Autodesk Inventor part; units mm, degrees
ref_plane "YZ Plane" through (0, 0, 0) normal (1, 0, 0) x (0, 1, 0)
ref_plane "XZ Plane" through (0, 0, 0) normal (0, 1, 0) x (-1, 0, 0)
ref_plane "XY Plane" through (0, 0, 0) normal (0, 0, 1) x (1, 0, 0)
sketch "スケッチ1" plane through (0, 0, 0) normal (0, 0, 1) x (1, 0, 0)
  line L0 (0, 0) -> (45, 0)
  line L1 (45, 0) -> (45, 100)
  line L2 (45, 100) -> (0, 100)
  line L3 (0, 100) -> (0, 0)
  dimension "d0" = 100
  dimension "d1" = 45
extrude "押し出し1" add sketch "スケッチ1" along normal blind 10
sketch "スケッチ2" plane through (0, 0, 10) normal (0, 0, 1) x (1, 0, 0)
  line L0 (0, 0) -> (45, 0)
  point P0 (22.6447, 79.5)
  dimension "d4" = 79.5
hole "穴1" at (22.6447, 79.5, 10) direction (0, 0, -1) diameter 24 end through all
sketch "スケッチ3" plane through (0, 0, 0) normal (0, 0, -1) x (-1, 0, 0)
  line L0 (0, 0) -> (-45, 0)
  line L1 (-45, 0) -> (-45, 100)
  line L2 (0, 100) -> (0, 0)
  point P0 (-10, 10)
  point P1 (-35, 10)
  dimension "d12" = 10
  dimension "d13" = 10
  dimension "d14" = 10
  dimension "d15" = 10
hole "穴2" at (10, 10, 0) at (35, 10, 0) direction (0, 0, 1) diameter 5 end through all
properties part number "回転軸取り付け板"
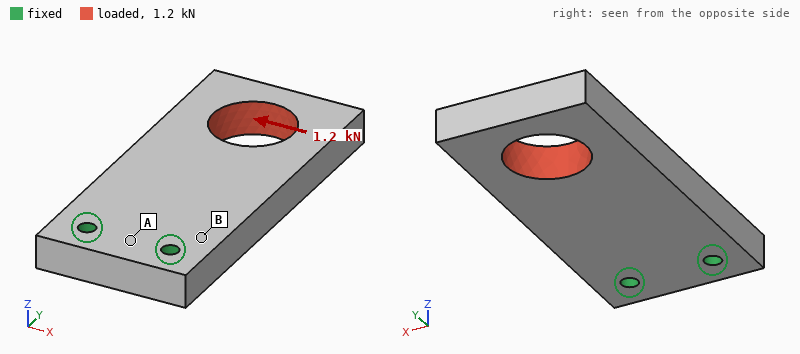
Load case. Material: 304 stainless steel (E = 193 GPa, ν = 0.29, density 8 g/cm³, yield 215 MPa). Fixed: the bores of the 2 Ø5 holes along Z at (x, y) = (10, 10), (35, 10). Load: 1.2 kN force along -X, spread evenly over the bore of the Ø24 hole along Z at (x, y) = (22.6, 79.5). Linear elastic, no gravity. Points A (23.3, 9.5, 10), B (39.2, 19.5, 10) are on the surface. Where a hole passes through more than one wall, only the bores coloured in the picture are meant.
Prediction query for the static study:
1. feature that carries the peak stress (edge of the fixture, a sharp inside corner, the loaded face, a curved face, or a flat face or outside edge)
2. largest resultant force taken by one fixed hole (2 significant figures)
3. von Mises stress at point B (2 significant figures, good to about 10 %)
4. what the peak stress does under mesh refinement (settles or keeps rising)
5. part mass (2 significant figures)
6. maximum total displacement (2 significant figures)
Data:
edge of the fixture
3.0 kN
17 MPa
keeps rising
320 g
23 µm
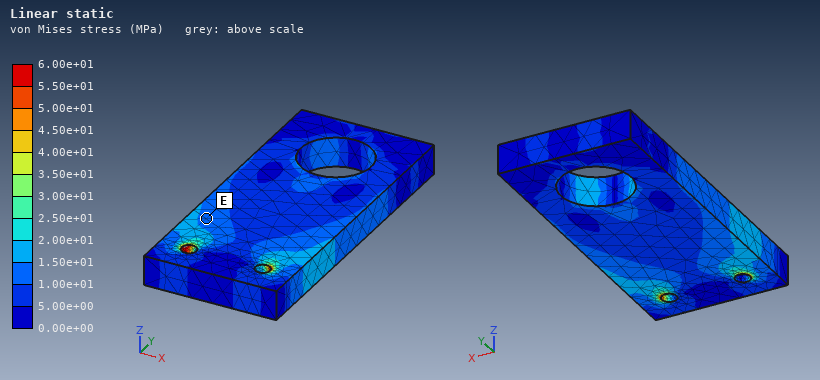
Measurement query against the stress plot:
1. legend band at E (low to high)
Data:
1.00e+01 to 1.50e+01 MPa
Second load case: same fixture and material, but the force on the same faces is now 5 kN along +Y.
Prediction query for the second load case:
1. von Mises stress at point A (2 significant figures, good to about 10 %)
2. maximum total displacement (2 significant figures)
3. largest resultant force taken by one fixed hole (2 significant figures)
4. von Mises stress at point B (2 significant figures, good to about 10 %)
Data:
3.6 MPa
8.1 µm
2.5 kN
13 MPa
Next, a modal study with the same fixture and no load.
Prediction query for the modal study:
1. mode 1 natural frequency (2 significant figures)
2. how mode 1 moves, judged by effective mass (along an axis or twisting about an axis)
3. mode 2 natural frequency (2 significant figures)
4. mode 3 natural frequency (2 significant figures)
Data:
1100 Hz
along Z
3700 Hz
3700 Hz
